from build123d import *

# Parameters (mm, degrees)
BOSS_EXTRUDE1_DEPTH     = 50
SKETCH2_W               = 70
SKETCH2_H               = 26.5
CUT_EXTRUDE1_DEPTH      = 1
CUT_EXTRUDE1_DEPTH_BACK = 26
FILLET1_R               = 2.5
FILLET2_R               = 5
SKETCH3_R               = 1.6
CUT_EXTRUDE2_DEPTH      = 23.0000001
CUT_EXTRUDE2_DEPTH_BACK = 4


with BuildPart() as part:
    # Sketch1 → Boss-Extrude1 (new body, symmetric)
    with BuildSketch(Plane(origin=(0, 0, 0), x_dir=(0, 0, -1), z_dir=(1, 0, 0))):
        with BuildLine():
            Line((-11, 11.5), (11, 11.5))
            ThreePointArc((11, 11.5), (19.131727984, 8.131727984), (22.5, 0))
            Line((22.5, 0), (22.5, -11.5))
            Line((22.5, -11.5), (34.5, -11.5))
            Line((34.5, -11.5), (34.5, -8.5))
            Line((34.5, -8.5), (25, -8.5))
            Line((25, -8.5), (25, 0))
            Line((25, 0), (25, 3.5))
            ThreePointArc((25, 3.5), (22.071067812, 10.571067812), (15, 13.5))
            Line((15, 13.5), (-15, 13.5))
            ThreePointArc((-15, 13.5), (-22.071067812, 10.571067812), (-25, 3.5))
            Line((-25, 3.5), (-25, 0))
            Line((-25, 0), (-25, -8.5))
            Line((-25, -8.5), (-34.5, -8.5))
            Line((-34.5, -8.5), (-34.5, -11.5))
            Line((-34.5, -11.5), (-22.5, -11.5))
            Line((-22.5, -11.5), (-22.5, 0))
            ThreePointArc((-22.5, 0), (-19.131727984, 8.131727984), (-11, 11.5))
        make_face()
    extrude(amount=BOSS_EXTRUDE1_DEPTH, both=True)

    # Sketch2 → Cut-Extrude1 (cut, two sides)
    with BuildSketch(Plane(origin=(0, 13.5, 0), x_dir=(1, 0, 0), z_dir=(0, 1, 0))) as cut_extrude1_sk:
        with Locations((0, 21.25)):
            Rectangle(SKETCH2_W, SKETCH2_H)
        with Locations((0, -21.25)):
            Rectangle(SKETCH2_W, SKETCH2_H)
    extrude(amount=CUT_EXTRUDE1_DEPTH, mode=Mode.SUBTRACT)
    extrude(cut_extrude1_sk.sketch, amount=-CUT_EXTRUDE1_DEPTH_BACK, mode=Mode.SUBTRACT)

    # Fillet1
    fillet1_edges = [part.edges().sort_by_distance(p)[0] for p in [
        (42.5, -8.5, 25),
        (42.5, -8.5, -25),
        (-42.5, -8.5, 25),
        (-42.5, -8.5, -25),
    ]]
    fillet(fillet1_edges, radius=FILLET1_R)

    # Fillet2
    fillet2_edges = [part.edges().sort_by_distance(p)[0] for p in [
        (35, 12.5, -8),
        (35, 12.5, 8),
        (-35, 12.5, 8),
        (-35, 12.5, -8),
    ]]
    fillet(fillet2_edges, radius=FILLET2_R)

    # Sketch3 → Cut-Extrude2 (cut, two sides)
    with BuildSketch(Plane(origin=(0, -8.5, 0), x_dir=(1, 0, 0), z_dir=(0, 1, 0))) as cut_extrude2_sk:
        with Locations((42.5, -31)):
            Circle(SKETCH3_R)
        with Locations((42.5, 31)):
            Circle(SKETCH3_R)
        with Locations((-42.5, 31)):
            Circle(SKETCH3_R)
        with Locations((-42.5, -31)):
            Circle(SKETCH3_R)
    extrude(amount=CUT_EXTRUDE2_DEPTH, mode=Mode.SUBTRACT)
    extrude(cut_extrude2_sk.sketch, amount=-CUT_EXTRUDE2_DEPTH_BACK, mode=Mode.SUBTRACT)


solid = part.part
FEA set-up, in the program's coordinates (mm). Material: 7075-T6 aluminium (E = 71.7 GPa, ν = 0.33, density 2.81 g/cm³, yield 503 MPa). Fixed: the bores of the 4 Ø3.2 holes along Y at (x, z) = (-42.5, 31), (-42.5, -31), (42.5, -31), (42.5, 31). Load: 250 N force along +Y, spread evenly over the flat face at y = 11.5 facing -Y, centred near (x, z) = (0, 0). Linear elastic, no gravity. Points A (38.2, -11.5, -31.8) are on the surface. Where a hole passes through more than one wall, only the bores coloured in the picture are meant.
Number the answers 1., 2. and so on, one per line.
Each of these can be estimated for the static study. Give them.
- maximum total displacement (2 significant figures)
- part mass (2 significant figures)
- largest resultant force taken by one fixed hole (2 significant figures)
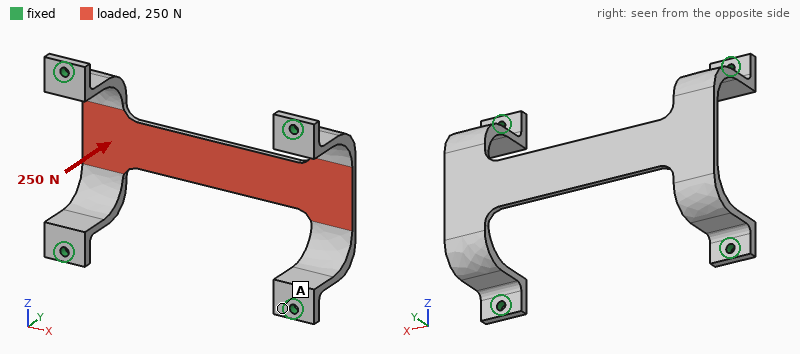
1. 0.37 mm
2. 30 g
3. 89 N
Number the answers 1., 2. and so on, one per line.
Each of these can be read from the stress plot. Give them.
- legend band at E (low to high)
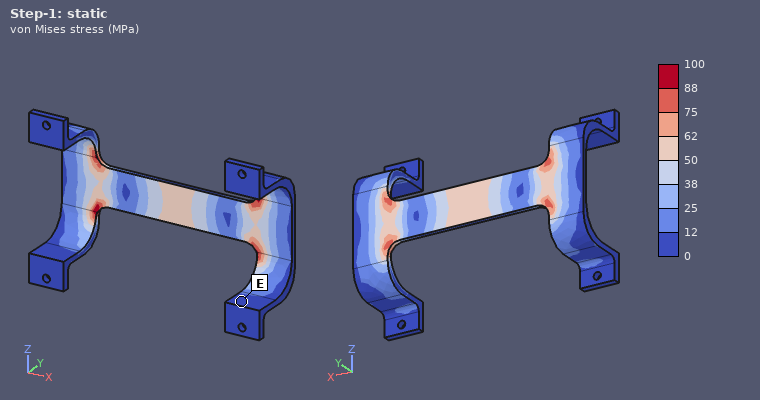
1. 0 to 12 MPa
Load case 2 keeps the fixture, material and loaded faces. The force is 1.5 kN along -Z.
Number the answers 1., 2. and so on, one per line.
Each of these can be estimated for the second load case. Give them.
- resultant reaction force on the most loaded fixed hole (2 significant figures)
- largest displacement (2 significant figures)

1. 420 N
2. 0.48 mm
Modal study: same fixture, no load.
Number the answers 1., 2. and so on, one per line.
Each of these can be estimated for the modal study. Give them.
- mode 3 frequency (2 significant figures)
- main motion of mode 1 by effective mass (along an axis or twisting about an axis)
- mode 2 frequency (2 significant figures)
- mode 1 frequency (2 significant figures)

1. 2500 Hz
2. along Y
3. 2500 Hz
4. 1500 Hz
